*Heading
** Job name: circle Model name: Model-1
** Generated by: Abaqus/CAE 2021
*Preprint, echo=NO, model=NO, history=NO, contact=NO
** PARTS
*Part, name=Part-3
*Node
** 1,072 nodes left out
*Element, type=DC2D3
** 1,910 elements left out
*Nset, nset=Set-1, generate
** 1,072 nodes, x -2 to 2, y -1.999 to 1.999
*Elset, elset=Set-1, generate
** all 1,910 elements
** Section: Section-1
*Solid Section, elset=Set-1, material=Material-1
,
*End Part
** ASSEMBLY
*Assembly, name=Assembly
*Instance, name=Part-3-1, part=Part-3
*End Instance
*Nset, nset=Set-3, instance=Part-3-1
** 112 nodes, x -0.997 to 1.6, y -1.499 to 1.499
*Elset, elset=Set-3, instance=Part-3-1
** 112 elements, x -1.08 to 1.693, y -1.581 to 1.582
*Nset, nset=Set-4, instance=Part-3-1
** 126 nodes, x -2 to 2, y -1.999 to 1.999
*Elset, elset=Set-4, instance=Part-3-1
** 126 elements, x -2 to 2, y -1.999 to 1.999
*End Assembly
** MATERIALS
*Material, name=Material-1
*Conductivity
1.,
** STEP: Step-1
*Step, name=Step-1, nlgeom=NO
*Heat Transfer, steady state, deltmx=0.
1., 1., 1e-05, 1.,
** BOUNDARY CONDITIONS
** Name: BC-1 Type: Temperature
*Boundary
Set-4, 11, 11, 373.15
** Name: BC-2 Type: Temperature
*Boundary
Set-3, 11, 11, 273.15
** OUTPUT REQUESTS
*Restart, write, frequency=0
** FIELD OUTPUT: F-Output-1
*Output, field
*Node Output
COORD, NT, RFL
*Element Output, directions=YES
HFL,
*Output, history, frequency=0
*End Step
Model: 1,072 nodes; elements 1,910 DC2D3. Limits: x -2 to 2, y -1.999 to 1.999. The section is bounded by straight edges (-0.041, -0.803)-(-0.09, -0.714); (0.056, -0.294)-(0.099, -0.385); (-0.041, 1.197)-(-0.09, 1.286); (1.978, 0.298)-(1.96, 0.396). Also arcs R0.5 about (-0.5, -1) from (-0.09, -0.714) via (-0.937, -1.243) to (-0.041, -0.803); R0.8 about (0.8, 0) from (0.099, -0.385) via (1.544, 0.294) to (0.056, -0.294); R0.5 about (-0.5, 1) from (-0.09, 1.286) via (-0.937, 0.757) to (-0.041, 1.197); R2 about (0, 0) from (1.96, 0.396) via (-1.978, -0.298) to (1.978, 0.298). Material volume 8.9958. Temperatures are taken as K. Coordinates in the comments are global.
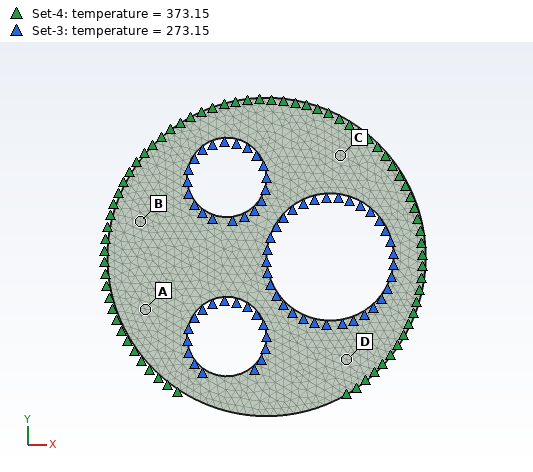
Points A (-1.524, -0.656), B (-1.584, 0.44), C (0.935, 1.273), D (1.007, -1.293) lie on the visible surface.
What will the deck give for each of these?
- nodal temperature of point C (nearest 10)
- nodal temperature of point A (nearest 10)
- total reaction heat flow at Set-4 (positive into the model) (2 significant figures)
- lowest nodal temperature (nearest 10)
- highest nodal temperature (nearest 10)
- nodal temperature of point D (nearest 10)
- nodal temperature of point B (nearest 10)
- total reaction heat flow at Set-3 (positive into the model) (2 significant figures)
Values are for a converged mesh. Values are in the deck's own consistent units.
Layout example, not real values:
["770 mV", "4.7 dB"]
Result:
["330 K", "340 K", "1700", "270 K", "370 K", "340 K", "350 K", "-1700"]
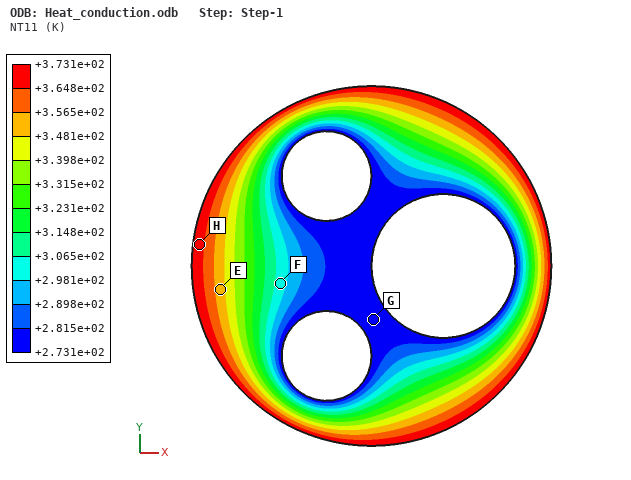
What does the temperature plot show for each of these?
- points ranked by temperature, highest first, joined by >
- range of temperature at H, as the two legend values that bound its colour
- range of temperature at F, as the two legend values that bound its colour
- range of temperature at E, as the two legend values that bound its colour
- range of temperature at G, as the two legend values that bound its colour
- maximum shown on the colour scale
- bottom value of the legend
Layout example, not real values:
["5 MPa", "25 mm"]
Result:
["H > E > F > G", "+3.648e+02 to +3.731e+02 K", "+2.981e+02 to +3.065e+02 K", "+3.481e+02 to +3.565e+02 K", "+2.731e+02 to +2.815e+02 K", "+3.731e+02 K", "+2.731e+02 K"]
